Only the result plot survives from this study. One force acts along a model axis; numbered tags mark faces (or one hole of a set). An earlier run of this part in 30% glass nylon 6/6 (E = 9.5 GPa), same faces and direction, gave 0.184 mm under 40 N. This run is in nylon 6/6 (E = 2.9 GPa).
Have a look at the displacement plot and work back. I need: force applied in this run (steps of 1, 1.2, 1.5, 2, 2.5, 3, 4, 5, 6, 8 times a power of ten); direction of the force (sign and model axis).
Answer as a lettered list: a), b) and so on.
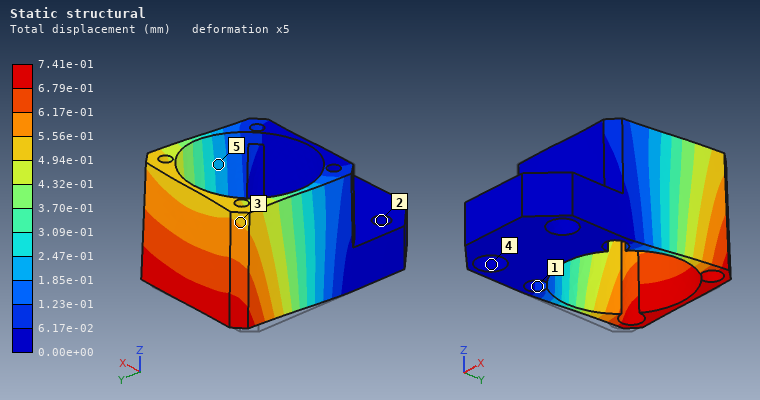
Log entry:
a) 50 N
b) +X
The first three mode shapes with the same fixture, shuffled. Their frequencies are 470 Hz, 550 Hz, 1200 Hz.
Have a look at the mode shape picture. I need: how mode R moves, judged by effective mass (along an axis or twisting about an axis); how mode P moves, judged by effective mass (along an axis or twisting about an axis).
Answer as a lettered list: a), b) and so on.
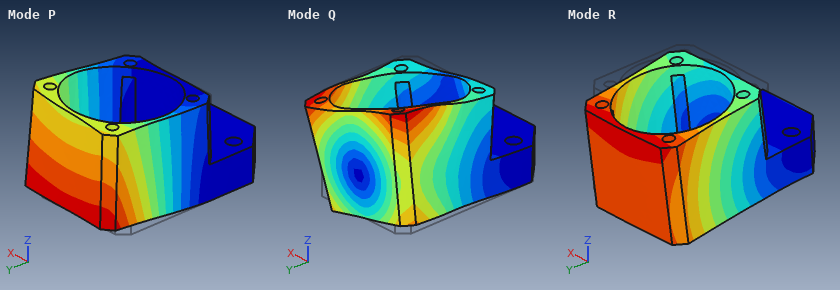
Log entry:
a) along Z
b) along X
